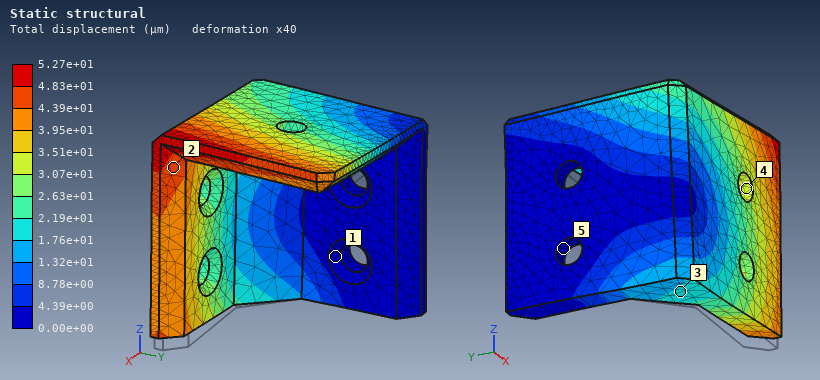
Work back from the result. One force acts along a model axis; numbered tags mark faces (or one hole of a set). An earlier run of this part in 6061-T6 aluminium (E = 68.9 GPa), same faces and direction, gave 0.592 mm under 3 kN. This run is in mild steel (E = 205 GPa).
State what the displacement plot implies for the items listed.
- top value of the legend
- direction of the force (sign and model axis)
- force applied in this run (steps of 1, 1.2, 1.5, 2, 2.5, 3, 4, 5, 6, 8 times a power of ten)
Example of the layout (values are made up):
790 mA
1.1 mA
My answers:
5.27e+01 µm
+Z
800 N
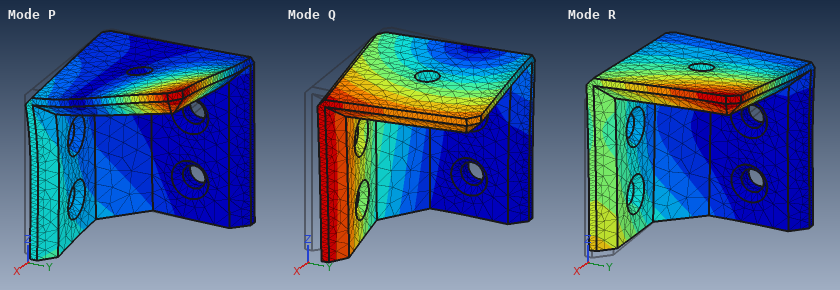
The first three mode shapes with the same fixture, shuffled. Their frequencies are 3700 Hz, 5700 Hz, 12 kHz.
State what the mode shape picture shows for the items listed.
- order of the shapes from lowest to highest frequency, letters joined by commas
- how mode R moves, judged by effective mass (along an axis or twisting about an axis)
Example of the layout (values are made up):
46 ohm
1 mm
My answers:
Q, R, P
along Z
